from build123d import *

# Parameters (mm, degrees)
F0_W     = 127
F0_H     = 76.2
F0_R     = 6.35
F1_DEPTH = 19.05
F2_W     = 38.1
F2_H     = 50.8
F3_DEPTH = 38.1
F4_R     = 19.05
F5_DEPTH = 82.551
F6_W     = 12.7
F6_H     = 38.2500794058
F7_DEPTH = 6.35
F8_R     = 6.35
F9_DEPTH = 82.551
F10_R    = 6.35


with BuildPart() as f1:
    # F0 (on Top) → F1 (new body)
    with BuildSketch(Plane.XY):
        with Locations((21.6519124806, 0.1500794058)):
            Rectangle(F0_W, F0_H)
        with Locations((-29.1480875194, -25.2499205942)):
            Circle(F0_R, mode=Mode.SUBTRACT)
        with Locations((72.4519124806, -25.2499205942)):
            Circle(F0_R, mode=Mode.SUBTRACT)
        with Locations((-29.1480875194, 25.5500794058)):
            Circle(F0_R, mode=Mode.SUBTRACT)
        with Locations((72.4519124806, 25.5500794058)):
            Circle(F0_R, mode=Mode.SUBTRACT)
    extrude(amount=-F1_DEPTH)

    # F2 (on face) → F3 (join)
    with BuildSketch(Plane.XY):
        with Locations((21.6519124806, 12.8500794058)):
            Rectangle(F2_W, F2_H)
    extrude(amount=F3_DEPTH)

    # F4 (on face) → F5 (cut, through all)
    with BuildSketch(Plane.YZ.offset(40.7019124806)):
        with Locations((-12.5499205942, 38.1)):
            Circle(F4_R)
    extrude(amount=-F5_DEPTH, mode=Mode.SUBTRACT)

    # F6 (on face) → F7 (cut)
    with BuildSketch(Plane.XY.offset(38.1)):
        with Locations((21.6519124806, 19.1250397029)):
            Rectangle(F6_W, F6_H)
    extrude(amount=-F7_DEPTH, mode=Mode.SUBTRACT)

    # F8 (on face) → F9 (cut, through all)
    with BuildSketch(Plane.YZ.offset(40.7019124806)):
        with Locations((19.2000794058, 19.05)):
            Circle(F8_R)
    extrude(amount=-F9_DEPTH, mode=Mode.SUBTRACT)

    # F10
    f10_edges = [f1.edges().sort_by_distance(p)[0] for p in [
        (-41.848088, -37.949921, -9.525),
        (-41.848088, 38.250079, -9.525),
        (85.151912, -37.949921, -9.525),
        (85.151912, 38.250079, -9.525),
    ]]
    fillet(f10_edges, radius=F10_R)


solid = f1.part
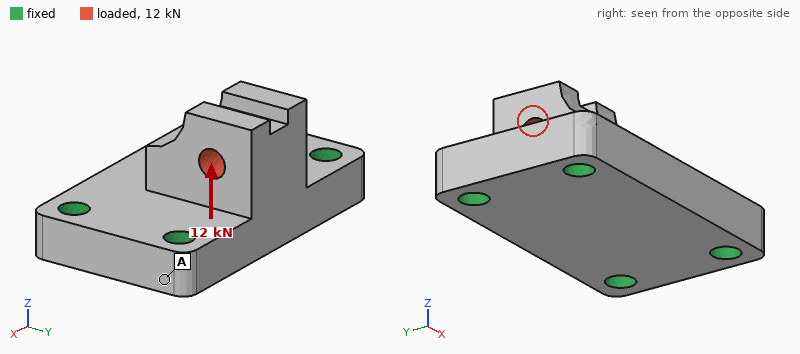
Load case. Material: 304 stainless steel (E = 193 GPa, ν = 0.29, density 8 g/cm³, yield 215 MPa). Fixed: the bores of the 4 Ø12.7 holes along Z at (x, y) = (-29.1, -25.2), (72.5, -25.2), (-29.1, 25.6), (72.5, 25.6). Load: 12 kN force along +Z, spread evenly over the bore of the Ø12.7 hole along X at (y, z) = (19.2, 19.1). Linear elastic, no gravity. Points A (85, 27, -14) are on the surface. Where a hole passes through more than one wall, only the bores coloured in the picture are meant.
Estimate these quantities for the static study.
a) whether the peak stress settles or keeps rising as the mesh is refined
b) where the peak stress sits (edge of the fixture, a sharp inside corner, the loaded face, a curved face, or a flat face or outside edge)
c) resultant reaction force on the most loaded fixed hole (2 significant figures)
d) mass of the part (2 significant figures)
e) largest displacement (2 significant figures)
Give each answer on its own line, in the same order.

keeps rising
edge of the fixture
5.1 kN
1.8 kg
14 µm
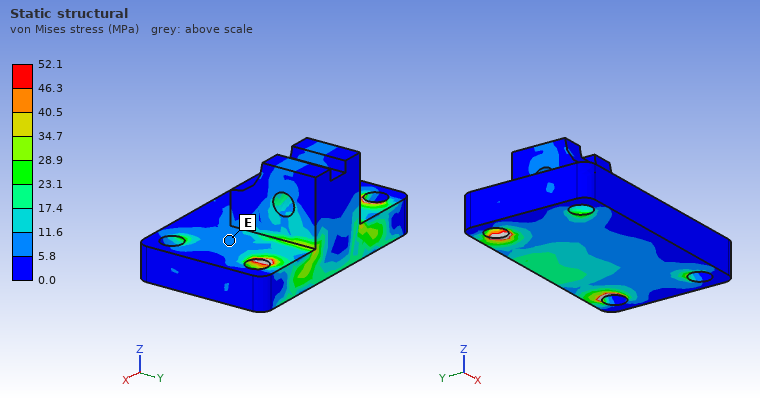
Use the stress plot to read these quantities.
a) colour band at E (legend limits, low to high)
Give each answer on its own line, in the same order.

5.8 to 11.6 MPa
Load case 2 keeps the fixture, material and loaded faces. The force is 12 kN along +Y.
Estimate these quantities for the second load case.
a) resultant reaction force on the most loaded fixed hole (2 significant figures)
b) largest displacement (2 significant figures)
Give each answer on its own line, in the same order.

5.0 kN
23 µm
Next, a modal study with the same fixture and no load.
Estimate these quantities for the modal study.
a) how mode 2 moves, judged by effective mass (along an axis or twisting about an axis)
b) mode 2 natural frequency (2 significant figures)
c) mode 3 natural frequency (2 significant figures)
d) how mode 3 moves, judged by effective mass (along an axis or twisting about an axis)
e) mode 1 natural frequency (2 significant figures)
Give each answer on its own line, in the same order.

along Z
7000 Hz
8600 Hz
along X
5900 Hz
